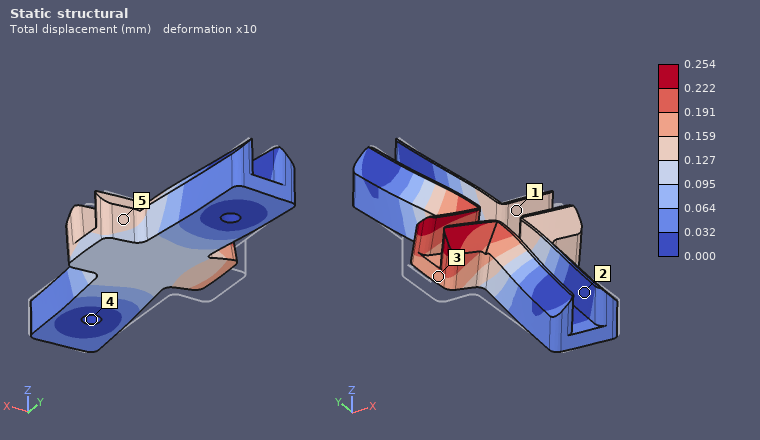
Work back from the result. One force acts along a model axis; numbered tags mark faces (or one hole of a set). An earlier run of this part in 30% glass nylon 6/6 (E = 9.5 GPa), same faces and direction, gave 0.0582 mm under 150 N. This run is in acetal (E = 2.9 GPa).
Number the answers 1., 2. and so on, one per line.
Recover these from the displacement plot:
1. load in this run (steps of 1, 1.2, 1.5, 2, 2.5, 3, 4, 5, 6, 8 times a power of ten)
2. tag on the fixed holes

1. 200 N
2. 4
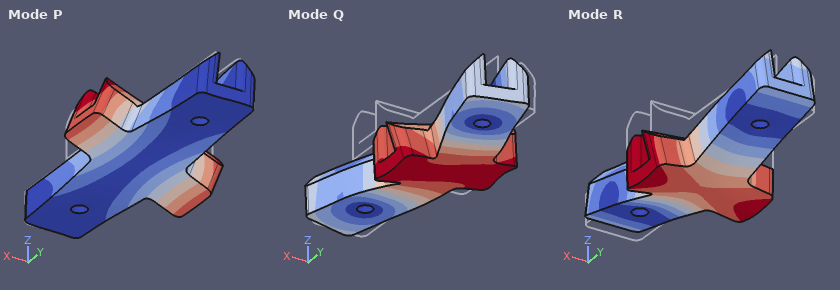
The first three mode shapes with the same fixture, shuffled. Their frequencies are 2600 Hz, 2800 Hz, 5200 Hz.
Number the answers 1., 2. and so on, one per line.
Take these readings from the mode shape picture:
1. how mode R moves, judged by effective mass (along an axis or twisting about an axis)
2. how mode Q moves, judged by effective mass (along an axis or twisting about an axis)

1. along Z
2. along X
